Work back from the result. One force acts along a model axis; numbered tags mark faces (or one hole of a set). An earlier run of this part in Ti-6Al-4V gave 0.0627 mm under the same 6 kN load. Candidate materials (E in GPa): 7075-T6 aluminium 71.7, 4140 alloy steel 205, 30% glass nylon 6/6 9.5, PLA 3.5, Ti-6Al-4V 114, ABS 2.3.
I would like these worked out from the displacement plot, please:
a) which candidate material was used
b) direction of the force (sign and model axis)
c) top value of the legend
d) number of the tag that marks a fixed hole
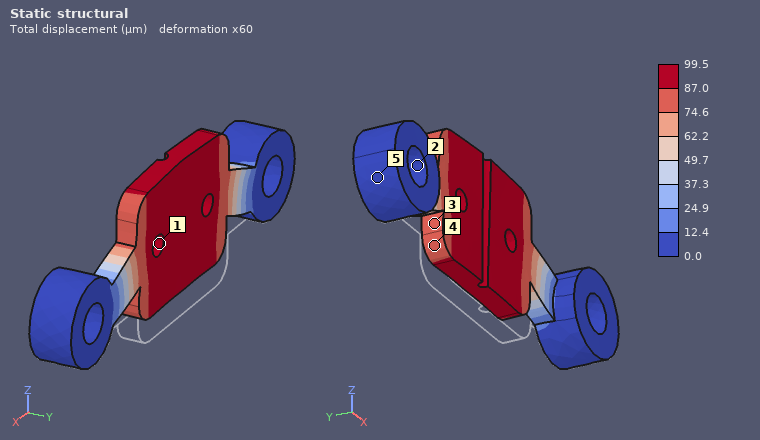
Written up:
7075-T6 aluminium
+Z
99.5 µm
2
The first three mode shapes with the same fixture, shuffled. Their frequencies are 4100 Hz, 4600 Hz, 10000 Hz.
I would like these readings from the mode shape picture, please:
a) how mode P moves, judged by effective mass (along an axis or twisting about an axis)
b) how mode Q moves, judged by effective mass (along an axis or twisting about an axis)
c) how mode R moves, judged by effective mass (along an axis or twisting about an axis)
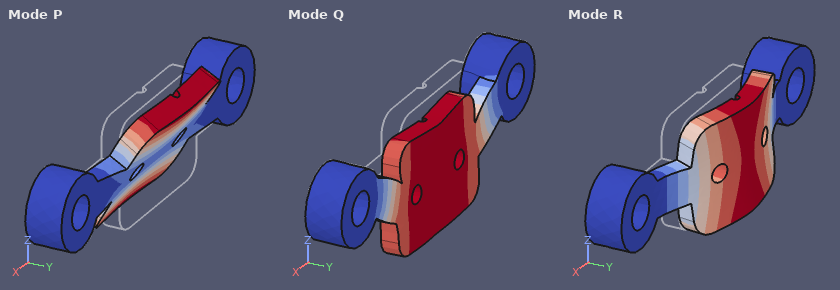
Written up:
twisting about X
along Z
along Y
